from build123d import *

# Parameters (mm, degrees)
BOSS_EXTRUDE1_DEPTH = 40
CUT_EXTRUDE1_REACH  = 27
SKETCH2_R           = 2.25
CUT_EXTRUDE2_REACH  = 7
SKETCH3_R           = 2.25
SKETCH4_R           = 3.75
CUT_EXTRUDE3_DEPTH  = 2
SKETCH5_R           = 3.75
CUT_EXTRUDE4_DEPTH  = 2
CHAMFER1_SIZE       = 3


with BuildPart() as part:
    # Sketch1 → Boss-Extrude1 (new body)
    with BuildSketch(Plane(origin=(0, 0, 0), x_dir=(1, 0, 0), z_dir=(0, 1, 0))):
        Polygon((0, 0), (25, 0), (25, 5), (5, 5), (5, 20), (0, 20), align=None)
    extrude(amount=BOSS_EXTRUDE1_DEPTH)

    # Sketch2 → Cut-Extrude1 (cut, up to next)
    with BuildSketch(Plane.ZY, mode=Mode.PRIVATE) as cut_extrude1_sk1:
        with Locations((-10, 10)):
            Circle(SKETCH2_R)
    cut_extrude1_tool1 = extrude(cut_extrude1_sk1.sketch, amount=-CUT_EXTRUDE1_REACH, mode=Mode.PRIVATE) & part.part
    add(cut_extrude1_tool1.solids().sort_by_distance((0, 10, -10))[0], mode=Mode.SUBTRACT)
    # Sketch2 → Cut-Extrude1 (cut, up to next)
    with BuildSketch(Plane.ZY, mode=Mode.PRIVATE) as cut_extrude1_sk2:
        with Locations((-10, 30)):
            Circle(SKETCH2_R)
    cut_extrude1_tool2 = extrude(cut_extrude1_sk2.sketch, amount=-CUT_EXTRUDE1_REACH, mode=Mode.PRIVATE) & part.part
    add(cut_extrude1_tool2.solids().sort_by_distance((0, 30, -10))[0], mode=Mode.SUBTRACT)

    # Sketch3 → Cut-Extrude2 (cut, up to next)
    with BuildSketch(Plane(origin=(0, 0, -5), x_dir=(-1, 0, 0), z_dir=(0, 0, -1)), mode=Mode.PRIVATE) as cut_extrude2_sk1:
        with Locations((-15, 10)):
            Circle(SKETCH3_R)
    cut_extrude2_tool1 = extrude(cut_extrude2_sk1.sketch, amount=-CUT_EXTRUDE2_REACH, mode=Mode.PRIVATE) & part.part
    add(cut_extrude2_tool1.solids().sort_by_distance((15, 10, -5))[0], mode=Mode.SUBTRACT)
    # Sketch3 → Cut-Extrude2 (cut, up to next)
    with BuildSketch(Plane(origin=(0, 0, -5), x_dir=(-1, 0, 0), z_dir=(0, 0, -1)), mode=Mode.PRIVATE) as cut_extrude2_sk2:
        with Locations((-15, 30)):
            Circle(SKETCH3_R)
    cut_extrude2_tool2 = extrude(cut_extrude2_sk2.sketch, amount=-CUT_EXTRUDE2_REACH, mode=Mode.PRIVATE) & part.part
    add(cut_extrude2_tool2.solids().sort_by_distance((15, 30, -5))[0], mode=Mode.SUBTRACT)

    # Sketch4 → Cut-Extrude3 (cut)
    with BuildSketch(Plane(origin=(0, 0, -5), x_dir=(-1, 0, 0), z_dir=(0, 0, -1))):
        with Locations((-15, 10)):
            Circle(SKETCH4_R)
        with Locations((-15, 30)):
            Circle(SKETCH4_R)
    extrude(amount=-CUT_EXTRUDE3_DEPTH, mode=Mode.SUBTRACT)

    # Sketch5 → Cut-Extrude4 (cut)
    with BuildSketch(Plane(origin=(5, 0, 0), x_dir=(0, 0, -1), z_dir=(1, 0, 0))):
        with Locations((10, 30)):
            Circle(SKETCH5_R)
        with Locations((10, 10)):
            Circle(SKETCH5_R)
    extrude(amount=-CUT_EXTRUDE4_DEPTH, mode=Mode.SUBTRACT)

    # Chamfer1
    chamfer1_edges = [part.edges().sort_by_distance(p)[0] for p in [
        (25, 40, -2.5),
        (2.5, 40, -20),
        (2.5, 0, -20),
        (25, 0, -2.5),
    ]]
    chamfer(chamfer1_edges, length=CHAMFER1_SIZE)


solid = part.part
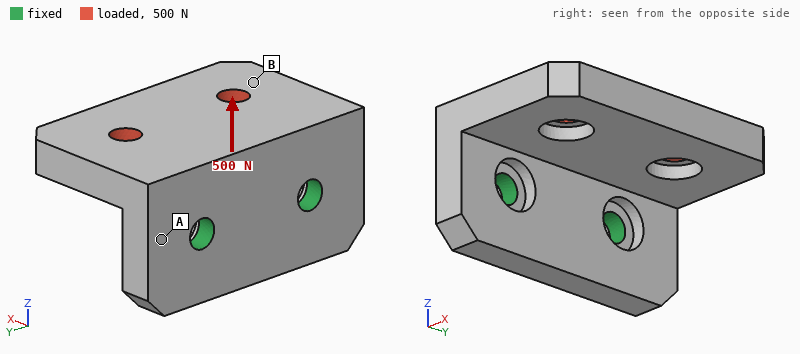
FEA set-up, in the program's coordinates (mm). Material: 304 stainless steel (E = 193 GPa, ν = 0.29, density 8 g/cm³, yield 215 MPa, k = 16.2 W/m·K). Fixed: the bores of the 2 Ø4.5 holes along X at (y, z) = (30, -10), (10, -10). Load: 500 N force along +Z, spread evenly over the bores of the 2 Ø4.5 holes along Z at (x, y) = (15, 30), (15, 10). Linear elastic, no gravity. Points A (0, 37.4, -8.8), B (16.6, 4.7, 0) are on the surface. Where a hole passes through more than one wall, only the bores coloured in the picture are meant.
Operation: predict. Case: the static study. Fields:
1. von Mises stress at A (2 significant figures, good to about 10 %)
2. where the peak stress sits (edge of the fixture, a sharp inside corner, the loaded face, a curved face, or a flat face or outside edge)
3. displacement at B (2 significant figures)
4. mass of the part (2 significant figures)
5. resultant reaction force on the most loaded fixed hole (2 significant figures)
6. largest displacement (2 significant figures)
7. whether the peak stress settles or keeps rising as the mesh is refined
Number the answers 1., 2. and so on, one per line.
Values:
1. 27 MPa
2. edge of the fixture
3. 20 µm
4. 59 g
5. 250 N
6. 31 µm
7. keeps rising
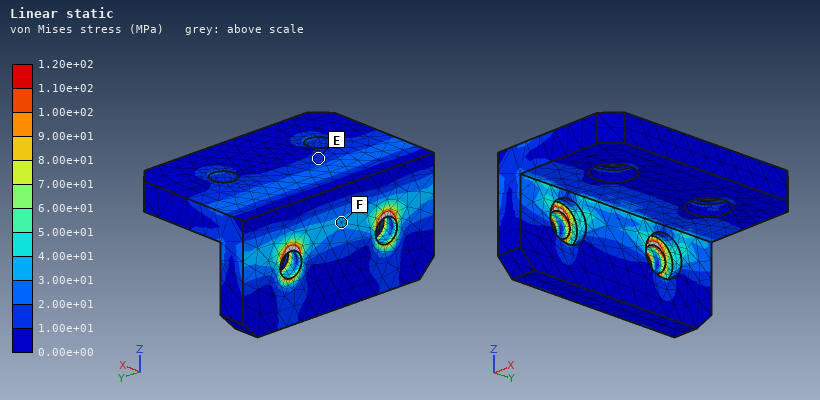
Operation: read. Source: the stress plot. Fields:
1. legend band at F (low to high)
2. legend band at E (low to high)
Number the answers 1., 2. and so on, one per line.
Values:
1. 3.00e+01 to 4.00e+01 MPa
2. 1.00e+01 to 2.00e+01 MPa
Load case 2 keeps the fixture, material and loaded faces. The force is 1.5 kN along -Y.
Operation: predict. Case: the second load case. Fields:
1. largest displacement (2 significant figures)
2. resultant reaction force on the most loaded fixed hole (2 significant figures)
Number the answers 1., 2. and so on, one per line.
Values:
1. 13 µm
2. 1.3 kN
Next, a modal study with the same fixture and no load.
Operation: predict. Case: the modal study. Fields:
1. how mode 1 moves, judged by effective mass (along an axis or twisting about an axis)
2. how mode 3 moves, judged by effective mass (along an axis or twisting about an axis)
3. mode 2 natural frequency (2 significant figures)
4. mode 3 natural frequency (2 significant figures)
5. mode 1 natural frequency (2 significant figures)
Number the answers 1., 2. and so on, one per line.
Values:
1. along Z
2. along Y
3. 8300 Hz
4. 13 kHz
5. 4300 Hz
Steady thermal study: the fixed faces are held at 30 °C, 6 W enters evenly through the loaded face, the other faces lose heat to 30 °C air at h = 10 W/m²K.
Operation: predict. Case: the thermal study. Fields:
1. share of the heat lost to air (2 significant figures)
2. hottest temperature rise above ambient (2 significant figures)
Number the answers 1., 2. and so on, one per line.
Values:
1. 13 %
2. 45 K
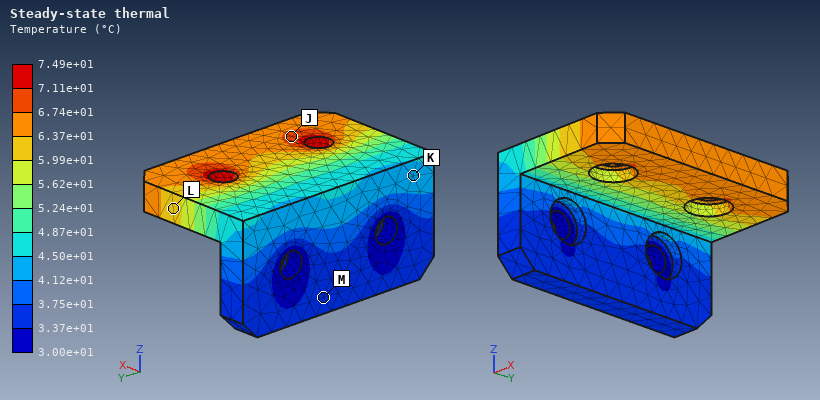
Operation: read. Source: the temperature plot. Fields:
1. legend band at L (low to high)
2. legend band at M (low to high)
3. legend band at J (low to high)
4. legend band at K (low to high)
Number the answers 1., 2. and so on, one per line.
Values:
1. 5.99e+01 to 6.37e+01 °C
2. 3.37e+01 to 3.75e+01 °C
3. 6.74e+01 to 7.11e+01 °C
4. 4.12e+01 to 4.50e+01 °C
